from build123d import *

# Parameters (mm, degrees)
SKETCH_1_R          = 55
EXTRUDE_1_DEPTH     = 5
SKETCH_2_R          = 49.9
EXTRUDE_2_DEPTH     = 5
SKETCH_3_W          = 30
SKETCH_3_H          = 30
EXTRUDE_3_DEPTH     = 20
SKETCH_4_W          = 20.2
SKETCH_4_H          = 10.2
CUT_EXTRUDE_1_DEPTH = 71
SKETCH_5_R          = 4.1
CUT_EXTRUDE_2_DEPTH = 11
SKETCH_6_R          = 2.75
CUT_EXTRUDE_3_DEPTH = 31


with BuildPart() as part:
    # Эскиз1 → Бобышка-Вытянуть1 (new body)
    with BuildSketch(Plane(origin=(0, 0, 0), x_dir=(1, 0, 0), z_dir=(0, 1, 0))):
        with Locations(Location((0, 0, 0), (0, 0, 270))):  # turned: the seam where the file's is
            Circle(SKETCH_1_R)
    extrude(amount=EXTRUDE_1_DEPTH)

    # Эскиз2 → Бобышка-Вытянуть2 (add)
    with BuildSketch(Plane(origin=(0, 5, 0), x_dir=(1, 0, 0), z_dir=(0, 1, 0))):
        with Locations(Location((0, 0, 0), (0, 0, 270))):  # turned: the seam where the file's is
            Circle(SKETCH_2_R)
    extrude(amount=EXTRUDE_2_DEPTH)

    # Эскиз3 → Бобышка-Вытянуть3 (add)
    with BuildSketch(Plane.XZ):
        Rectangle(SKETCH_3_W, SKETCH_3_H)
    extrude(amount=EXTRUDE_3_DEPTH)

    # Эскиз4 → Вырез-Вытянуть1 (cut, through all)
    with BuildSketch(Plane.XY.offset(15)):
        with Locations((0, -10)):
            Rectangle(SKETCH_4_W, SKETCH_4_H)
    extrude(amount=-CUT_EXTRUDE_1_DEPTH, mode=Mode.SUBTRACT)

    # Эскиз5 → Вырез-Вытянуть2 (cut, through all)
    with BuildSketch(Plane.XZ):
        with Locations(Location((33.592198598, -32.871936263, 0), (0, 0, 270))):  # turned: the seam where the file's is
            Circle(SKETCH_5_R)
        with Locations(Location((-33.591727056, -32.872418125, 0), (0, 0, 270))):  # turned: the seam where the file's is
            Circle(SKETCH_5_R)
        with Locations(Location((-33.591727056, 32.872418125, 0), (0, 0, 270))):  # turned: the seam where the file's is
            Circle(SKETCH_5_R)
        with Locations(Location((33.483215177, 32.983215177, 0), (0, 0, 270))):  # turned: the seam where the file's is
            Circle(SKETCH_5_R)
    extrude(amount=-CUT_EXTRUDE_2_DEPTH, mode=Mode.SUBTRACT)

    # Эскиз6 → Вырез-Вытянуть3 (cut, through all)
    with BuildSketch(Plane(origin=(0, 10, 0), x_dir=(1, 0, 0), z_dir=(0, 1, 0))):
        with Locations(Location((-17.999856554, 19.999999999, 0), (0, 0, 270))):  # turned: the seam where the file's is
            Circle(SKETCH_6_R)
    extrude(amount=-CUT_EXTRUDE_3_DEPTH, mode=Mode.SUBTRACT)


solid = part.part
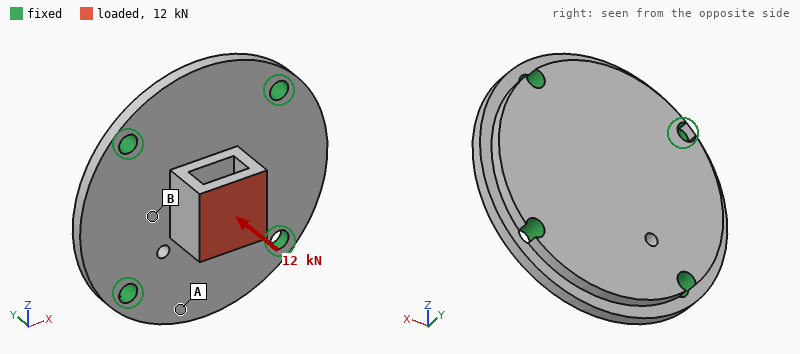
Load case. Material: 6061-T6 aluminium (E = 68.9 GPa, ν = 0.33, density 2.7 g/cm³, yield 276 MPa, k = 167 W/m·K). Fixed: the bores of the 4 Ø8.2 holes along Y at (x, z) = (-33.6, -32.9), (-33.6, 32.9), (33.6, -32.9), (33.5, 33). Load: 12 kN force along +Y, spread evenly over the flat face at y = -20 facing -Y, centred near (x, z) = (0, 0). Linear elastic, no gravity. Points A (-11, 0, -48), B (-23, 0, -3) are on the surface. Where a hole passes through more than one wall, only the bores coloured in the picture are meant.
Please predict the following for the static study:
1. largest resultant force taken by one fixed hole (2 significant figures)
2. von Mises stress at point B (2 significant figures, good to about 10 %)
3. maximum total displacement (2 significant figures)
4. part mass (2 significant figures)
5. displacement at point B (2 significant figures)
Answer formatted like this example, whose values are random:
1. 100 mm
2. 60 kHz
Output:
1. 3.1 kN
2. 34 MPa
3. 0.10 mm
4. 260 g
5. 0.047 mm
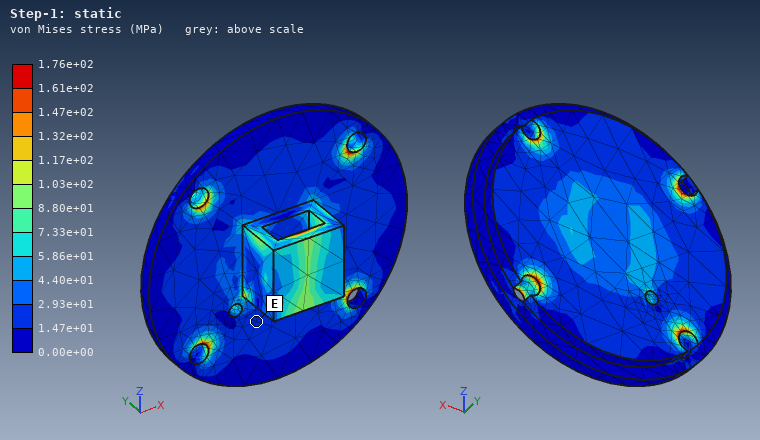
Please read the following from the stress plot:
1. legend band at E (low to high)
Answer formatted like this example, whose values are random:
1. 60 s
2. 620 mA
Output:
1. 1.47e+01 to 2.93e+01 MPa
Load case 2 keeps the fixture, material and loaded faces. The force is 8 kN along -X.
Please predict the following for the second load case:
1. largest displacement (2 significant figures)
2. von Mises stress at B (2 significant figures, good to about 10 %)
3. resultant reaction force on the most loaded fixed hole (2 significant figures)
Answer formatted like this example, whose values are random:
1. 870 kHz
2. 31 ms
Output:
1. 0.14 mm
2. 35 MPa
3. 2.8 kN
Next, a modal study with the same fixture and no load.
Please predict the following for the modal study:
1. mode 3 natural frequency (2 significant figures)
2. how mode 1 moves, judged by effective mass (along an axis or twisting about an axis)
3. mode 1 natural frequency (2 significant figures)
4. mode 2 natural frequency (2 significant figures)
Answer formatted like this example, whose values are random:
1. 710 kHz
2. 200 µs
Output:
1. 9000 Hz
2. along Y
3. 7100 Hz
4. 9000 Hz
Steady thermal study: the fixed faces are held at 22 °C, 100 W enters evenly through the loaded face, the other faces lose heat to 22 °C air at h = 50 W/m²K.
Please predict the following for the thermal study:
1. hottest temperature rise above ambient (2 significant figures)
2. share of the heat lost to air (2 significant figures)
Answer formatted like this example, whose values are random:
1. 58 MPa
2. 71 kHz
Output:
1. 54 K
2. 12 %
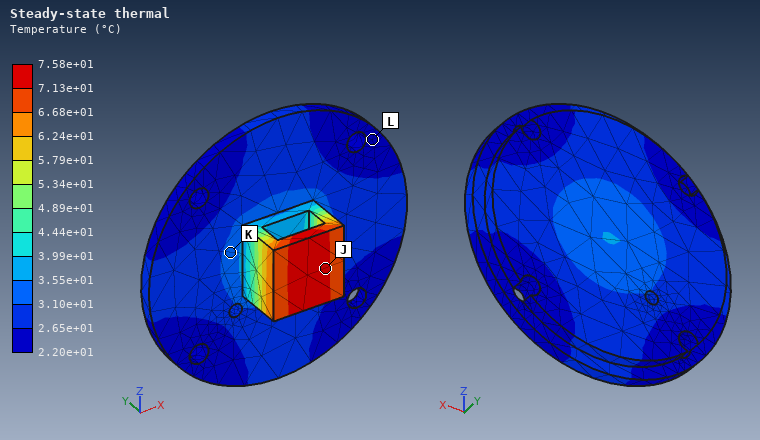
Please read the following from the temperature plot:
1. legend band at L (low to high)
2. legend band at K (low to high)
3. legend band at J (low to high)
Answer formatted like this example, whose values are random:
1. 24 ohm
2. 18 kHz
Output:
1. 2.20e+01 to 2.65e+01 °C
2. 3.10e+01 to 3.55e+01 °C
3. 7.13e+01 to 7.58e+01 °C
